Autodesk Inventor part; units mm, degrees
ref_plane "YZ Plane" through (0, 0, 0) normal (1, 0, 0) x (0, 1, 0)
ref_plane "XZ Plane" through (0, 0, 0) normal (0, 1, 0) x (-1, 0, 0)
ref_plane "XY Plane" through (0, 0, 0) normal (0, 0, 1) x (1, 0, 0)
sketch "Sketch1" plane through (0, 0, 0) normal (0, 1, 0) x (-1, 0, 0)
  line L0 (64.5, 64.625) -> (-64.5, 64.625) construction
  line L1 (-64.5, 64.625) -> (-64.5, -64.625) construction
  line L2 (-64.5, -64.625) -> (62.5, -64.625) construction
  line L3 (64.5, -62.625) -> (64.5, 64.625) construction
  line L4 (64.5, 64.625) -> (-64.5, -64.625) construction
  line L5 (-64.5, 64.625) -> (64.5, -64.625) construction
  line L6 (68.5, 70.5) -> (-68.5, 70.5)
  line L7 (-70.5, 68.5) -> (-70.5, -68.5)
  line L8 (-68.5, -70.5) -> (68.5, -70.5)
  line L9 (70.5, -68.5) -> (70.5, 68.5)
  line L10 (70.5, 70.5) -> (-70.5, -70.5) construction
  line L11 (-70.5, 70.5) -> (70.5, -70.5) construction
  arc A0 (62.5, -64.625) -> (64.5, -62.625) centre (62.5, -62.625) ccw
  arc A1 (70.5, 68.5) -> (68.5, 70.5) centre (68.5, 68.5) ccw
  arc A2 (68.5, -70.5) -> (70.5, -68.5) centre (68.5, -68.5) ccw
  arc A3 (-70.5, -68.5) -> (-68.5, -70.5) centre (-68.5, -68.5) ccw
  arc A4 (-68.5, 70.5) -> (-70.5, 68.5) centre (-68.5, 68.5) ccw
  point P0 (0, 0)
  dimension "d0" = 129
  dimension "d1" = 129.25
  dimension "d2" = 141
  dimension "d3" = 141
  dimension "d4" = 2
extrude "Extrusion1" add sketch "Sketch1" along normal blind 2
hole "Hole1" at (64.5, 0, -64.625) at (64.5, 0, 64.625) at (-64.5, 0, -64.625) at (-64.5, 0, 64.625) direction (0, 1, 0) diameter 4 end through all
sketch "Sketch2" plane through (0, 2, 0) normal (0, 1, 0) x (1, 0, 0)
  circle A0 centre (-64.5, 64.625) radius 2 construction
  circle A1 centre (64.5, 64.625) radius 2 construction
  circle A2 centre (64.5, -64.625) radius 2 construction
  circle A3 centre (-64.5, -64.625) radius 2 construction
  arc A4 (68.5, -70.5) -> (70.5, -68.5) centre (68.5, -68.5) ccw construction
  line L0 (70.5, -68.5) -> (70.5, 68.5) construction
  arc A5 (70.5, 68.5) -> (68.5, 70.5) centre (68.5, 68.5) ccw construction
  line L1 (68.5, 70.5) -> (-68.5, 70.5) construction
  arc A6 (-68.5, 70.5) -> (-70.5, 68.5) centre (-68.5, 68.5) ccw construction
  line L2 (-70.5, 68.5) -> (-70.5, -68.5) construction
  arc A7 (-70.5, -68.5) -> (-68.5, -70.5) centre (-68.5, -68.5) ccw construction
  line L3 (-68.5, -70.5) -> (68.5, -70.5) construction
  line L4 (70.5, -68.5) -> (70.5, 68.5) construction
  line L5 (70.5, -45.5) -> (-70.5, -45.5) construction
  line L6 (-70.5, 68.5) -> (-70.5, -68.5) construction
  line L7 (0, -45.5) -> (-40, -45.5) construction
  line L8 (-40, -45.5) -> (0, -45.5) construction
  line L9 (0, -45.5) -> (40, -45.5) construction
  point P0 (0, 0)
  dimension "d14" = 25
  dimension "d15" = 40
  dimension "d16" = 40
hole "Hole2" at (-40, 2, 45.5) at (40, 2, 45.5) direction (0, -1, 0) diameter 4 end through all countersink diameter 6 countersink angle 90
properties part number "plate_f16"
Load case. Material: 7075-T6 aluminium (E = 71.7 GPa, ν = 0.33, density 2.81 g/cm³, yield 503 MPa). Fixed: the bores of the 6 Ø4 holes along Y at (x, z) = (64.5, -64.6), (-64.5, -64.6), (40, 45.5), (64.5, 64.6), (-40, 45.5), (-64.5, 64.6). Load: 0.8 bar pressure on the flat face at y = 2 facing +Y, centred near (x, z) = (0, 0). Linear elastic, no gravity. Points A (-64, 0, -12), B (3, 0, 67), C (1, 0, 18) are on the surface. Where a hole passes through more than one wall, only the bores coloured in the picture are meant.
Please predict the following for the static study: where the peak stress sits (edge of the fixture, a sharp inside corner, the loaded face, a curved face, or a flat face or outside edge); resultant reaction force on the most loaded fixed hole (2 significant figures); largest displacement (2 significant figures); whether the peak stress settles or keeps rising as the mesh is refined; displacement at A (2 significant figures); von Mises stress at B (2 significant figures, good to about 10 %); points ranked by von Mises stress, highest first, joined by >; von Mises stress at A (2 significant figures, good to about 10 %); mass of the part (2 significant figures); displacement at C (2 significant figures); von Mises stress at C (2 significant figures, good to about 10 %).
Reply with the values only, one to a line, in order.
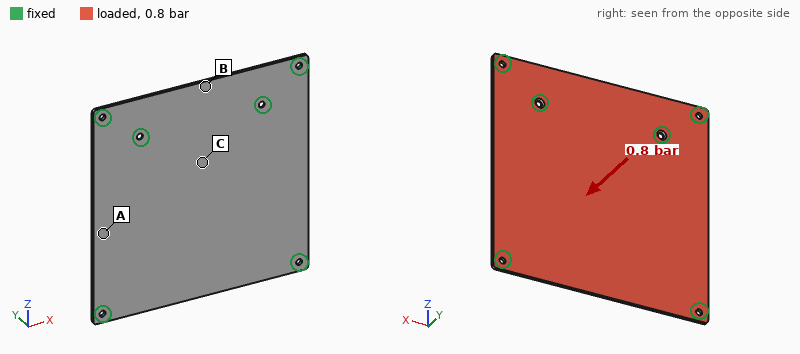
edge of the fixture
590 N
1.8 mm
keeps rising
0.95 mm
25 MPa
A > C > B
85 MPa
110 g
1.0 mm
45 MPa
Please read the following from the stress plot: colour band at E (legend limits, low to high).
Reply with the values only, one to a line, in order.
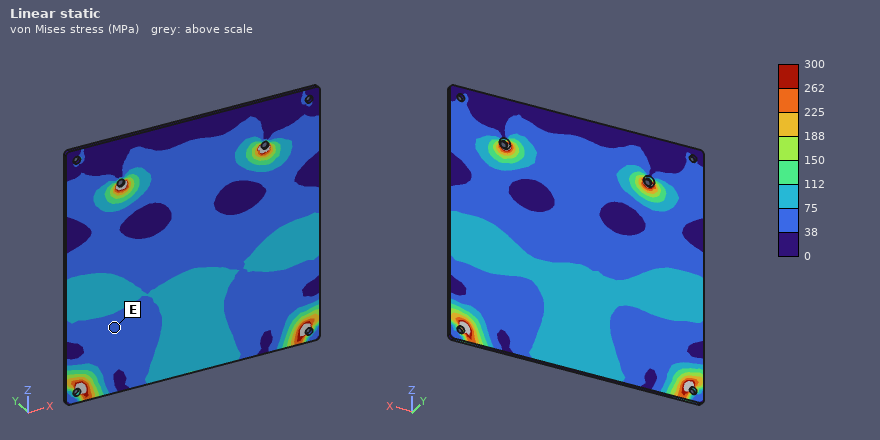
38 to 75 MPa
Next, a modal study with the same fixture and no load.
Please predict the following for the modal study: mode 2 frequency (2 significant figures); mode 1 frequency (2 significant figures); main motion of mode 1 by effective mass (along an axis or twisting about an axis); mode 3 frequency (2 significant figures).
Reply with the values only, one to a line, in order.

830 Hz
520 Hz
along Y
830 Hz
